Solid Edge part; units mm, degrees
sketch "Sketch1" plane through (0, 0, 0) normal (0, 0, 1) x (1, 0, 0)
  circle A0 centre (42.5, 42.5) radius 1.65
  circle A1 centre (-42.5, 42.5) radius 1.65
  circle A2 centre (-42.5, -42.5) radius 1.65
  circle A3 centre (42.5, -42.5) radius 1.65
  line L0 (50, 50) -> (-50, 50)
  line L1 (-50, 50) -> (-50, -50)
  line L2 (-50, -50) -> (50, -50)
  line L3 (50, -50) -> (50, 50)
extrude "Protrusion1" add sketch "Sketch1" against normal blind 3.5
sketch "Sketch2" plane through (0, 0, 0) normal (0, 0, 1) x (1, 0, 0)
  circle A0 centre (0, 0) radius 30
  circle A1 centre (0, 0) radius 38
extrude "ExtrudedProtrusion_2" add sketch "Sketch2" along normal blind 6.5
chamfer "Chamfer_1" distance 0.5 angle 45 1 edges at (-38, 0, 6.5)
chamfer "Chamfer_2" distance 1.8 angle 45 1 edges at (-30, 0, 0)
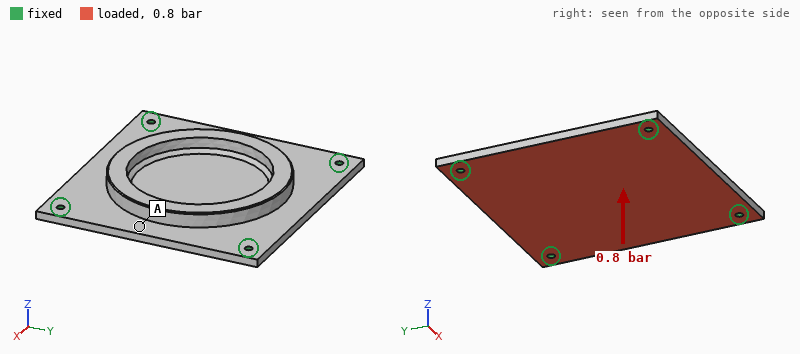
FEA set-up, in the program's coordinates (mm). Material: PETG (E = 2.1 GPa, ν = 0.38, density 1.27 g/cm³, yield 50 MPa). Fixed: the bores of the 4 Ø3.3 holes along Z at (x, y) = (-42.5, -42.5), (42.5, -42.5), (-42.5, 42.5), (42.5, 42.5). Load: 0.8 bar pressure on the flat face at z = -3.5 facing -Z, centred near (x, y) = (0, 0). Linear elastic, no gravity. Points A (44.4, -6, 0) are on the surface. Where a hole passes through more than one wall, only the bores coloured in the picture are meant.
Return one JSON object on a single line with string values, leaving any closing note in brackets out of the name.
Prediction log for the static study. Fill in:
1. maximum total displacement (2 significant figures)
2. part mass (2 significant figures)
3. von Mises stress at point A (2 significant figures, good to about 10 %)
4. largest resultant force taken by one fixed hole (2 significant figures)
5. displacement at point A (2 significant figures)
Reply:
{"maximum total displacement": "1.7 mm", "part mass": "59 g", "von Mises stress at point A": "5.9 MPa", "largest resultant force taken by one fixed hole": "220 N", "displacement at point A": "1.2 mm"}
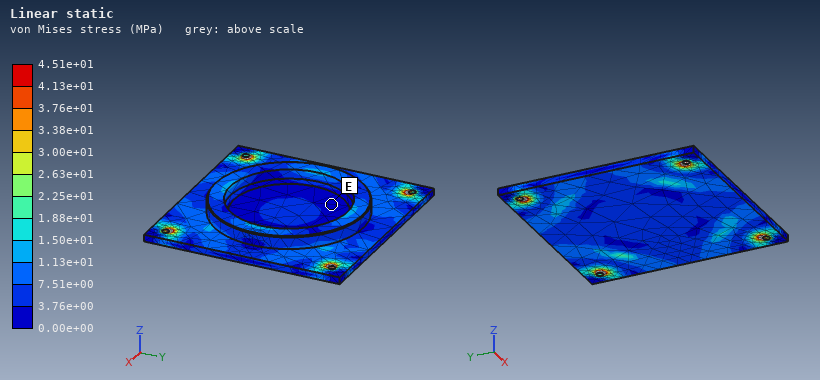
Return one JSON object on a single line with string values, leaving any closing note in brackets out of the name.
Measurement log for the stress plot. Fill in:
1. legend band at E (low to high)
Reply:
{"legend band at E": "0.00e+00 to 3.76e+00 MPa"}
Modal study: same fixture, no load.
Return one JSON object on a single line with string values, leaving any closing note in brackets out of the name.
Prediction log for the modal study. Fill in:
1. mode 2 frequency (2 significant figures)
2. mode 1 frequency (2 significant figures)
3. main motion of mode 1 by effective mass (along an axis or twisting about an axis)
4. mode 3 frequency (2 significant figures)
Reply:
{"mode 2 frequency": "770 Hz", "mode 1 frequency": "510 Hz", "main motion of mode 1 by effective mass": "along Z", "mode 3 frequency": "770 Hz"}
